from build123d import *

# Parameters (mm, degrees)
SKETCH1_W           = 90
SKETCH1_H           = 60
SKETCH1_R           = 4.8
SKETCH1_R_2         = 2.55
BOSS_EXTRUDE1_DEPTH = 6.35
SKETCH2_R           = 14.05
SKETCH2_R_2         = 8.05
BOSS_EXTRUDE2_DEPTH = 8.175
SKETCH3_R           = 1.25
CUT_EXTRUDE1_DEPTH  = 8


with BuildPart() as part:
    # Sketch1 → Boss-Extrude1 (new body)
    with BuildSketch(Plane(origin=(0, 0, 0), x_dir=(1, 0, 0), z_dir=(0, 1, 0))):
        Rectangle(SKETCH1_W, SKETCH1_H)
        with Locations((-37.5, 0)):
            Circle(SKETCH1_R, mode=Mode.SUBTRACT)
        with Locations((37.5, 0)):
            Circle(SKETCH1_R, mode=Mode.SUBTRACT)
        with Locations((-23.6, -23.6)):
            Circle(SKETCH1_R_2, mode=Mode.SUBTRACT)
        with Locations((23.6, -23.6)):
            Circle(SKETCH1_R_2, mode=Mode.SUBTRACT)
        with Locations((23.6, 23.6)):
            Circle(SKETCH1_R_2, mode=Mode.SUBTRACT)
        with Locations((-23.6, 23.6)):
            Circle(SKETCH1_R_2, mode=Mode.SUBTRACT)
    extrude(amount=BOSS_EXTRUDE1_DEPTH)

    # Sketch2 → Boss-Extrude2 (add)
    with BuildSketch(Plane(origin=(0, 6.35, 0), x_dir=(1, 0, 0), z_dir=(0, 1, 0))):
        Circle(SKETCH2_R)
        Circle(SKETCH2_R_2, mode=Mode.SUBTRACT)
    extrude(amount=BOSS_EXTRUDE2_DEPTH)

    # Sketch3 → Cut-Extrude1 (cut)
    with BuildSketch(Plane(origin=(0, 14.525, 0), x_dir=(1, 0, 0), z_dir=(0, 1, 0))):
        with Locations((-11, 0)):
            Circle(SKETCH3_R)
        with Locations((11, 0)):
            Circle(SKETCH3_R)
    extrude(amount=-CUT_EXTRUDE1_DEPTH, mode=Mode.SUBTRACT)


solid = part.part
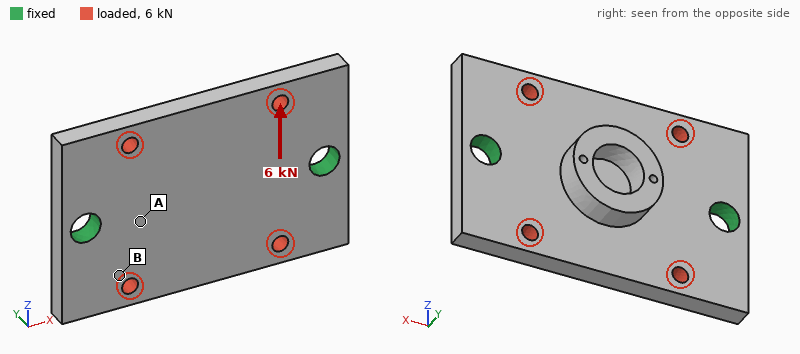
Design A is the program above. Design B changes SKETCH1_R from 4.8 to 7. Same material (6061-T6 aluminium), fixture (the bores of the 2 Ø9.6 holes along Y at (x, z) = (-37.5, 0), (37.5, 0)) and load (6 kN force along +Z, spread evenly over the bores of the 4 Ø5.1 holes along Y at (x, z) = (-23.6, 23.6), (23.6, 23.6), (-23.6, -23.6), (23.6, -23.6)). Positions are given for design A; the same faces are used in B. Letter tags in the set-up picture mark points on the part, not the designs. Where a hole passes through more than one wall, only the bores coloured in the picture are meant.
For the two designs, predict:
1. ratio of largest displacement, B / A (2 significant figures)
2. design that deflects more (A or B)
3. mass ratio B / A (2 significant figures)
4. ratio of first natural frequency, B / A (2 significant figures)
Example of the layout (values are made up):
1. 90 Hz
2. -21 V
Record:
1. 0.86
2. A
3. 0.97
4. 1.2
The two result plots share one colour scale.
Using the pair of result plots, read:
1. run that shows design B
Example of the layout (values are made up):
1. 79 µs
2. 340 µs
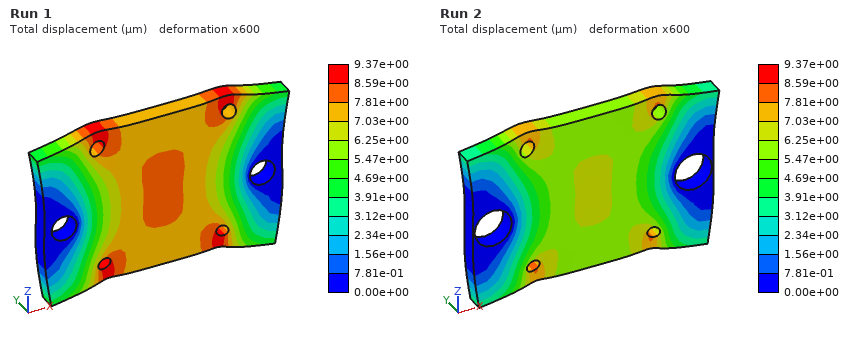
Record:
1. Run 2
